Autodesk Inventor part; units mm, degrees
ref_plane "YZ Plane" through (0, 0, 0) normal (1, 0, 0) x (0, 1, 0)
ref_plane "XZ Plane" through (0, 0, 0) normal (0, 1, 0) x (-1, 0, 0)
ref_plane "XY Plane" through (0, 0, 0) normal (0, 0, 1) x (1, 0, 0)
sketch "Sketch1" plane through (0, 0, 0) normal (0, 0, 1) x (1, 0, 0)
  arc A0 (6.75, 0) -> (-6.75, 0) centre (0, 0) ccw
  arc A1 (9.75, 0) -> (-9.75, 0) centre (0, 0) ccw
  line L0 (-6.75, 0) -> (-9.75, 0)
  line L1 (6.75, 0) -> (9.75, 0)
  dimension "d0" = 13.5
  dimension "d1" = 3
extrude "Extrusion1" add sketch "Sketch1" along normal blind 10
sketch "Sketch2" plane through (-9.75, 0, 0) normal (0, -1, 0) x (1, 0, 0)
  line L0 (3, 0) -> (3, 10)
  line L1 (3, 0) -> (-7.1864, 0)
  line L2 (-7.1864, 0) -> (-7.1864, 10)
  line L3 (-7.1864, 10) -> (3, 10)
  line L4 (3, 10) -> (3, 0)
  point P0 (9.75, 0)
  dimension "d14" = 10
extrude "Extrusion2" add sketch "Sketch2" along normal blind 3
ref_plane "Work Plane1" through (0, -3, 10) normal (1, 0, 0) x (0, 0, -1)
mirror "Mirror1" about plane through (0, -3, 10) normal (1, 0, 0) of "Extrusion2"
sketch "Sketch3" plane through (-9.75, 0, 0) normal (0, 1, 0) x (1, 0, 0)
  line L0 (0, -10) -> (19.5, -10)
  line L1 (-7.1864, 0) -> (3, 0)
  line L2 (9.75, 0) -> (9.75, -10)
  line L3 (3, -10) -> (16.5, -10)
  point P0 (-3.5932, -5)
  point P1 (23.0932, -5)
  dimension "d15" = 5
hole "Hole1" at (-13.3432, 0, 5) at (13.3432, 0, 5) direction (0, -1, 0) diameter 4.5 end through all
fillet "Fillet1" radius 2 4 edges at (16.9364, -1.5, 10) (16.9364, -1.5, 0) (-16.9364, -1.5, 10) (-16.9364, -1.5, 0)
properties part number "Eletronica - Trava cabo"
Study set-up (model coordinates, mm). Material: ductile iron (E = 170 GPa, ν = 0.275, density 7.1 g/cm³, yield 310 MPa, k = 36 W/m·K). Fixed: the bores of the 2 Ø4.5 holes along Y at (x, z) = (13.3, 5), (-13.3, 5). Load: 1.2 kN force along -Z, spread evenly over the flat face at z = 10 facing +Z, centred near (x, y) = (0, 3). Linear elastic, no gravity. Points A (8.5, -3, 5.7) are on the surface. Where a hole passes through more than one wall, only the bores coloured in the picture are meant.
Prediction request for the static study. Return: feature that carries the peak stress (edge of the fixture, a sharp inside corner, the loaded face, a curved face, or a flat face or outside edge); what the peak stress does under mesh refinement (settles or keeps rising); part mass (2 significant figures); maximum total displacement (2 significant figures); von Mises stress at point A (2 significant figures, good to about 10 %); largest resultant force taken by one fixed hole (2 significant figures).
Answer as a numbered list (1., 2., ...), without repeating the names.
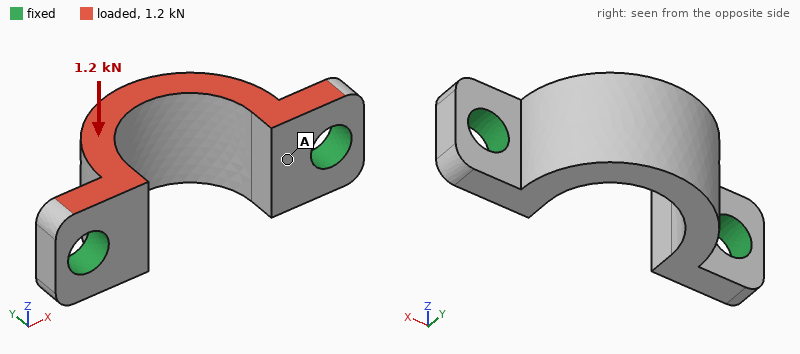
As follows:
1. edge of the fixture
2. keeps rising
3. 9.1 g
4. 19 µm
5. 30 MPa
6. 600 N
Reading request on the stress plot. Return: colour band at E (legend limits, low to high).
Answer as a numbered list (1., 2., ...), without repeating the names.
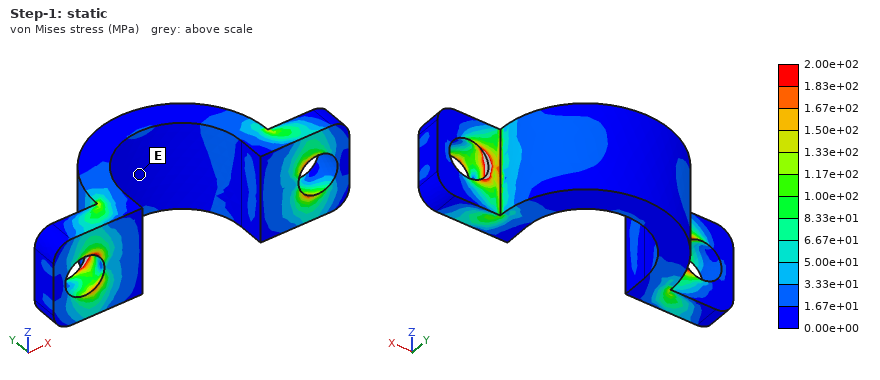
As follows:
1. 0.00e+00 to 1.67e+01 MPa
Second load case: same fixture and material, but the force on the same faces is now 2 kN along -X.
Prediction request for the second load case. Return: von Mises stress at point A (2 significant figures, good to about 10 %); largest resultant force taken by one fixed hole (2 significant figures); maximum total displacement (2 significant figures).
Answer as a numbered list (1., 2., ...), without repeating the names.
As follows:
1. 63 MPa
2. 1.1 kN
3. 18 µm
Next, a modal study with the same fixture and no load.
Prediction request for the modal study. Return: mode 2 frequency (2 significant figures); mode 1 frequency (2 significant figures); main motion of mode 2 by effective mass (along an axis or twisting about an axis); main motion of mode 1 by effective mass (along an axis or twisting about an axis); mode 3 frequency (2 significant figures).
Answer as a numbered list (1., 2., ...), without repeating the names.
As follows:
1. 25 kHz
2. 16 kHz
3. along X
4. along Z
5. 35 kHz
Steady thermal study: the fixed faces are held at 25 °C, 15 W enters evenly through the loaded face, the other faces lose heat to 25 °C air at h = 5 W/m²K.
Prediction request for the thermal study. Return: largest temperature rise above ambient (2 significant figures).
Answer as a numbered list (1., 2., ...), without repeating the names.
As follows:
1. 60 K
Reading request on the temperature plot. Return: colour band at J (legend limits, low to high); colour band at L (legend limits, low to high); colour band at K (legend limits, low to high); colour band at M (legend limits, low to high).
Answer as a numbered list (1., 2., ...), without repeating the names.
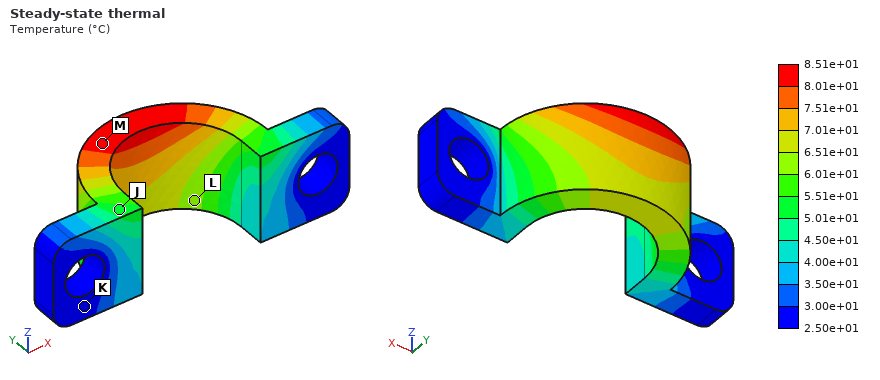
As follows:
1. 5.01e+01 to 5.51e+01 °C
2. 6.01e+01 to 6.51e+01 °C
3. 2.50e+01 to 3.00e+01 °C
4. 8.01e+01 to 8.51e+01 °C
